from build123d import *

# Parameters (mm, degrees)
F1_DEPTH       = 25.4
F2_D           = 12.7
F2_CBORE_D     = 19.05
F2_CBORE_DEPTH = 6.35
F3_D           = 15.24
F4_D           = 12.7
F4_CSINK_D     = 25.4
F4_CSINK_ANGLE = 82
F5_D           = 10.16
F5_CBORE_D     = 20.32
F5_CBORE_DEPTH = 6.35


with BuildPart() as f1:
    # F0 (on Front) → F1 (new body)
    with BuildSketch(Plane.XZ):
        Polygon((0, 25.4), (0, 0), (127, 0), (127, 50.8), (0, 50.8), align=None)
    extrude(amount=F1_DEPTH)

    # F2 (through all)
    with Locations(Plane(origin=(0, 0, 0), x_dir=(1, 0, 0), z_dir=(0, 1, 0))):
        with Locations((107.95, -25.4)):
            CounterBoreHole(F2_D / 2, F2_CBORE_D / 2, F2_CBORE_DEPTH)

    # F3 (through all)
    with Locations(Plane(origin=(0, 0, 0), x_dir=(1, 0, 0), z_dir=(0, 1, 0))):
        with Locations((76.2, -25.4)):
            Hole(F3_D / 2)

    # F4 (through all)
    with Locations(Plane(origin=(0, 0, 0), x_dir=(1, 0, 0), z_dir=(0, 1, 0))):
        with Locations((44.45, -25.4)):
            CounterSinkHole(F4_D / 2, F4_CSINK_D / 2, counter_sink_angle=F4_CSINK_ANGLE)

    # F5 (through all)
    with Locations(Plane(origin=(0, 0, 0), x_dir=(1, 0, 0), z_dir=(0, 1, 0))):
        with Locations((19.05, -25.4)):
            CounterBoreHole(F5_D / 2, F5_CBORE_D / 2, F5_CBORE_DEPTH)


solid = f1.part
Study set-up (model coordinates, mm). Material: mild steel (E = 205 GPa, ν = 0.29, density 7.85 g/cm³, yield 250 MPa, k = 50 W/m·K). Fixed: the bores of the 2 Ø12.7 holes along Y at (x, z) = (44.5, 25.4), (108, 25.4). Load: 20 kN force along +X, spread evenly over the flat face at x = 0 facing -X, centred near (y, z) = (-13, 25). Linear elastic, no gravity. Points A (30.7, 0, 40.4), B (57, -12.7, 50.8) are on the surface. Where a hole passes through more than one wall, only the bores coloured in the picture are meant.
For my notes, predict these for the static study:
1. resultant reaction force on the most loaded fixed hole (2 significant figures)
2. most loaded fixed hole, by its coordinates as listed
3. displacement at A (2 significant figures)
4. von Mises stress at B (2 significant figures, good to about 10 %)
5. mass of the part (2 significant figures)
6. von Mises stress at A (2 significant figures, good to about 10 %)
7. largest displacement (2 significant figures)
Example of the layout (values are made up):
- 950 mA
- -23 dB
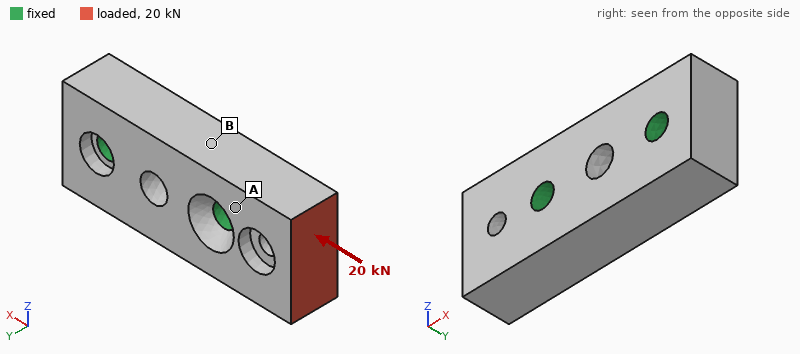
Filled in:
- 17 kN
- (44.5, 25.4)
- 3.2 µm
- 9.1 MPa
- 1.2 kg
- 22 MPa
- 8.5 µm
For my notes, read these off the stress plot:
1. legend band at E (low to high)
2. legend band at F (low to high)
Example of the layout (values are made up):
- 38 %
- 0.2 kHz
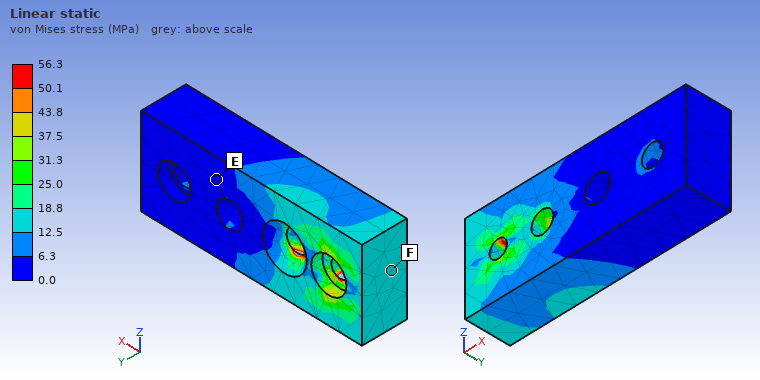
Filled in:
- 0.0 to 6.3 MPa
- 12.5 to 18.8 MPa
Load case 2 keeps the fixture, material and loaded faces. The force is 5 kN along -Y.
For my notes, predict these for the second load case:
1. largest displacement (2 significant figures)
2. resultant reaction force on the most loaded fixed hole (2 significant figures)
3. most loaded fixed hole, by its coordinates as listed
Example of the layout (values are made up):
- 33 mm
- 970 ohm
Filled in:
- 21 µm
- 6.4 kN
- (44.5, 25.4)
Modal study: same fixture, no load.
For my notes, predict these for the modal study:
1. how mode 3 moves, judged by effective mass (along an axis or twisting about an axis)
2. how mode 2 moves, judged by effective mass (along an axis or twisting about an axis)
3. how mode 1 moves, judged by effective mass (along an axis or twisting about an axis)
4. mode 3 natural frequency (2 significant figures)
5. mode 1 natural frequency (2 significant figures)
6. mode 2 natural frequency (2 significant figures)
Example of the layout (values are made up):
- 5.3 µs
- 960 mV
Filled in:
- twisting about X
- along Z
- along Y
- 10 kHz
- 7200 Hz
- 8800 Hz
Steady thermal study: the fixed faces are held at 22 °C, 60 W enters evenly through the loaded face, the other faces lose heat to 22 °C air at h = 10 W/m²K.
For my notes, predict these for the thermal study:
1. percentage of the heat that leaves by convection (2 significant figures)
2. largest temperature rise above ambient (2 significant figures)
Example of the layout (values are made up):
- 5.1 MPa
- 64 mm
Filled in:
- 3.7 %
- 50 K
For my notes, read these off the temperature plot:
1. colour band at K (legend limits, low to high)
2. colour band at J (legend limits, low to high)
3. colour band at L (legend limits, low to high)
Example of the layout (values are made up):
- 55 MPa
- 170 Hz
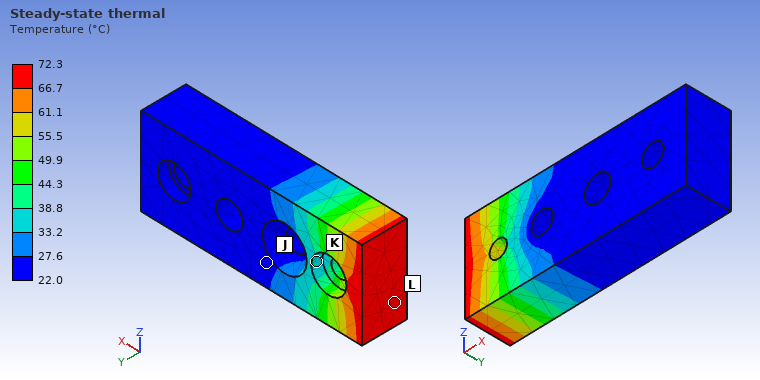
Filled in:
- 33.2 to 38.8 °C
- 22.0 to 27.6 °C
- 66.7 to 72.3 °C
